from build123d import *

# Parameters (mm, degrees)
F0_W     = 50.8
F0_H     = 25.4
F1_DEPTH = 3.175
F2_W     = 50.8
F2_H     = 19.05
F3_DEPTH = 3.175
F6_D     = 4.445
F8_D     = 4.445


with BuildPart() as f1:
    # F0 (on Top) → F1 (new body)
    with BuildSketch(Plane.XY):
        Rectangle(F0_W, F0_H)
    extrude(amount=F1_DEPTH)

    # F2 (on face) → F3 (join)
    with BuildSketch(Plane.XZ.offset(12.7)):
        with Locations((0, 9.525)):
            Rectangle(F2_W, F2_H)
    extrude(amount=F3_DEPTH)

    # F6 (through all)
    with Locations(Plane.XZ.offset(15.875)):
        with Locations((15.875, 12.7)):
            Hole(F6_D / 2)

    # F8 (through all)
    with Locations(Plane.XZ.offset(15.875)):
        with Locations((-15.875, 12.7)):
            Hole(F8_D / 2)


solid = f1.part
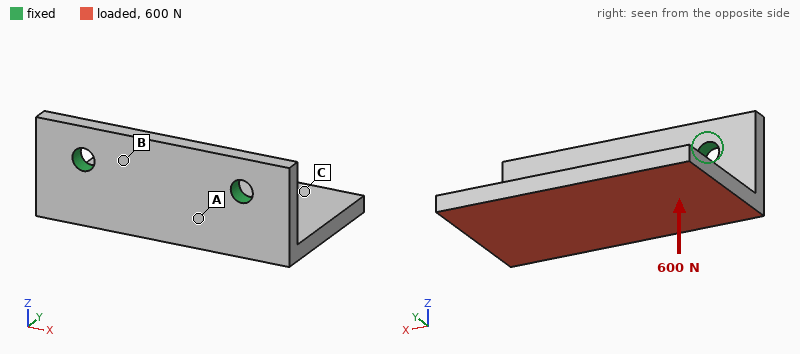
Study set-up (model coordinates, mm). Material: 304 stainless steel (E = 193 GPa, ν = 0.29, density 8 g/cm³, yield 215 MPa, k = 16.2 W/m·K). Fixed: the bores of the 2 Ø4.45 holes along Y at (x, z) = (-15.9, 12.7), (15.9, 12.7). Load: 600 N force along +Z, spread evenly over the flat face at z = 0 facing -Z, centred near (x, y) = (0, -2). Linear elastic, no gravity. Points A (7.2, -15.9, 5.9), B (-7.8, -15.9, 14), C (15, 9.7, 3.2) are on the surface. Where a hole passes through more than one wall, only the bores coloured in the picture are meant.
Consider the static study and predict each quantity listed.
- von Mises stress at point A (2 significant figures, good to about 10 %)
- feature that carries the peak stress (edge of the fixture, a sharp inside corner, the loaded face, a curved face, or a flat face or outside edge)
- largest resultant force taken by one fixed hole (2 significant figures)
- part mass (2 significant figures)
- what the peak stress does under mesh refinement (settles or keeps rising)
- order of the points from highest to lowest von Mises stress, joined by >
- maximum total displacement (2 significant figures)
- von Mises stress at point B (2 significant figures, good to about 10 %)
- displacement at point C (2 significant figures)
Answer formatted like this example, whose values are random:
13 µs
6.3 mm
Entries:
72 MPa
edge of the fixture
310 N
57 g
keeps rising
A > B > C
0.13 mm
29 MPa
0.11 mm
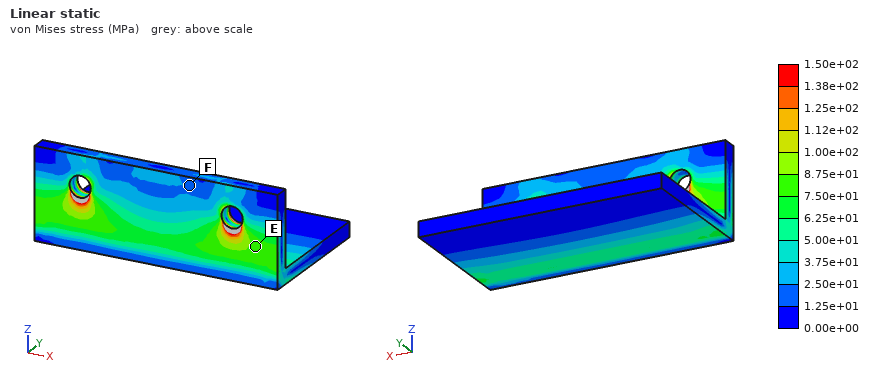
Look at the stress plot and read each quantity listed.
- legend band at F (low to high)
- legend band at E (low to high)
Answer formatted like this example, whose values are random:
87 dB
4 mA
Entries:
1.25e+01 to 2.50e+01 MPa
7.50e+01 to 8.75e+01 MPa
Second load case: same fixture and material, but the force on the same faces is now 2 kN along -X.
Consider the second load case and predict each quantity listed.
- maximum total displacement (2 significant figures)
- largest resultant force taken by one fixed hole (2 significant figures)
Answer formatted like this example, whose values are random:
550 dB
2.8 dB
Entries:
45 µm
1.4 kN
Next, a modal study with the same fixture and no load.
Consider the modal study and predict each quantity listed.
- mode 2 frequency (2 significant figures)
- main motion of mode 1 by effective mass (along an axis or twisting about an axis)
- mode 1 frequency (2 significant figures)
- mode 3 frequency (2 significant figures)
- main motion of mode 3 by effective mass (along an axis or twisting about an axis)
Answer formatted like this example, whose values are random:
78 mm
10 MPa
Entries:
4100 Hz
along Z
2100 Hz
6900 Hz
along X
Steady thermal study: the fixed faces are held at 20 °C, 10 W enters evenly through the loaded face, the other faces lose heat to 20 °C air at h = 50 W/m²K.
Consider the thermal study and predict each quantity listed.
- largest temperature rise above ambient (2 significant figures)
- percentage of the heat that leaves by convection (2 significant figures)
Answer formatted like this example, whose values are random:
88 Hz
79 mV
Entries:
53 K
49 %
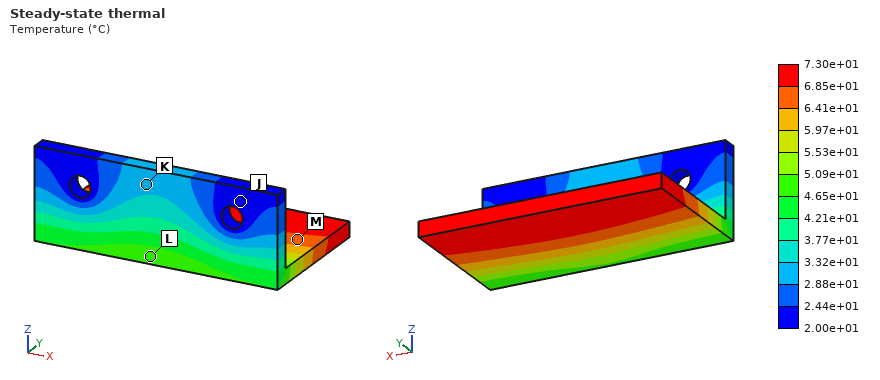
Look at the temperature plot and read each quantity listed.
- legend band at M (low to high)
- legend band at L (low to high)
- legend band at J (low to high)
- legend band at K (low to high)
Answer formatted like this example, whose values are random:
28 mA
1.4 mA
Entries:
6.41e+01 to 6.85e+01 °C
4.65e+01 to 5.09e+01 °C
2.00e+01 to 2.44e+01 °C
2.88e+01 to 3.32e+01 °C
